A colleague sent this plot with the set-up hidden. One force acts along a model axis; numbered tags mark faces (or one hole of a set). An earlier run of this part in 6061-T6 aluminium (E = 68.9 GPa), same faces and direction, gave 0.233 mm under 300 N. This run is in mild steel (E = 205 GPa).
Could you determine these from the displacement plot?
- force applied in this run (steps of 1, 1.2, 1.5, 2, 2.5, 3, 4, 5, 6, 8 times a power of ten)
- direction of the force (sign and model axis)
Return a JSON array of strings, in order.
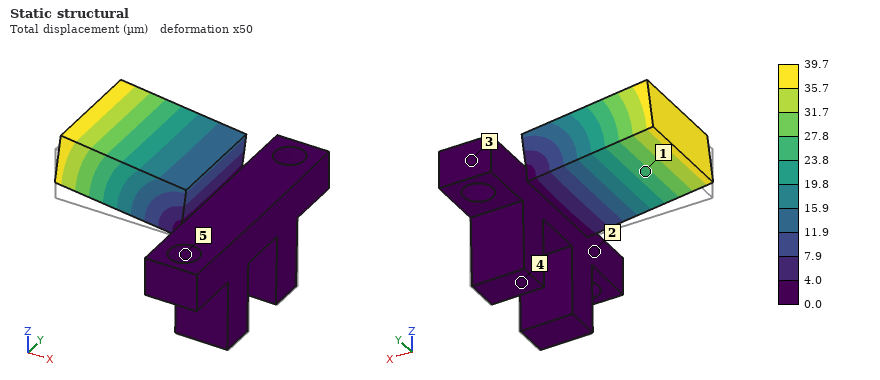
["150 N", "+Z"]
